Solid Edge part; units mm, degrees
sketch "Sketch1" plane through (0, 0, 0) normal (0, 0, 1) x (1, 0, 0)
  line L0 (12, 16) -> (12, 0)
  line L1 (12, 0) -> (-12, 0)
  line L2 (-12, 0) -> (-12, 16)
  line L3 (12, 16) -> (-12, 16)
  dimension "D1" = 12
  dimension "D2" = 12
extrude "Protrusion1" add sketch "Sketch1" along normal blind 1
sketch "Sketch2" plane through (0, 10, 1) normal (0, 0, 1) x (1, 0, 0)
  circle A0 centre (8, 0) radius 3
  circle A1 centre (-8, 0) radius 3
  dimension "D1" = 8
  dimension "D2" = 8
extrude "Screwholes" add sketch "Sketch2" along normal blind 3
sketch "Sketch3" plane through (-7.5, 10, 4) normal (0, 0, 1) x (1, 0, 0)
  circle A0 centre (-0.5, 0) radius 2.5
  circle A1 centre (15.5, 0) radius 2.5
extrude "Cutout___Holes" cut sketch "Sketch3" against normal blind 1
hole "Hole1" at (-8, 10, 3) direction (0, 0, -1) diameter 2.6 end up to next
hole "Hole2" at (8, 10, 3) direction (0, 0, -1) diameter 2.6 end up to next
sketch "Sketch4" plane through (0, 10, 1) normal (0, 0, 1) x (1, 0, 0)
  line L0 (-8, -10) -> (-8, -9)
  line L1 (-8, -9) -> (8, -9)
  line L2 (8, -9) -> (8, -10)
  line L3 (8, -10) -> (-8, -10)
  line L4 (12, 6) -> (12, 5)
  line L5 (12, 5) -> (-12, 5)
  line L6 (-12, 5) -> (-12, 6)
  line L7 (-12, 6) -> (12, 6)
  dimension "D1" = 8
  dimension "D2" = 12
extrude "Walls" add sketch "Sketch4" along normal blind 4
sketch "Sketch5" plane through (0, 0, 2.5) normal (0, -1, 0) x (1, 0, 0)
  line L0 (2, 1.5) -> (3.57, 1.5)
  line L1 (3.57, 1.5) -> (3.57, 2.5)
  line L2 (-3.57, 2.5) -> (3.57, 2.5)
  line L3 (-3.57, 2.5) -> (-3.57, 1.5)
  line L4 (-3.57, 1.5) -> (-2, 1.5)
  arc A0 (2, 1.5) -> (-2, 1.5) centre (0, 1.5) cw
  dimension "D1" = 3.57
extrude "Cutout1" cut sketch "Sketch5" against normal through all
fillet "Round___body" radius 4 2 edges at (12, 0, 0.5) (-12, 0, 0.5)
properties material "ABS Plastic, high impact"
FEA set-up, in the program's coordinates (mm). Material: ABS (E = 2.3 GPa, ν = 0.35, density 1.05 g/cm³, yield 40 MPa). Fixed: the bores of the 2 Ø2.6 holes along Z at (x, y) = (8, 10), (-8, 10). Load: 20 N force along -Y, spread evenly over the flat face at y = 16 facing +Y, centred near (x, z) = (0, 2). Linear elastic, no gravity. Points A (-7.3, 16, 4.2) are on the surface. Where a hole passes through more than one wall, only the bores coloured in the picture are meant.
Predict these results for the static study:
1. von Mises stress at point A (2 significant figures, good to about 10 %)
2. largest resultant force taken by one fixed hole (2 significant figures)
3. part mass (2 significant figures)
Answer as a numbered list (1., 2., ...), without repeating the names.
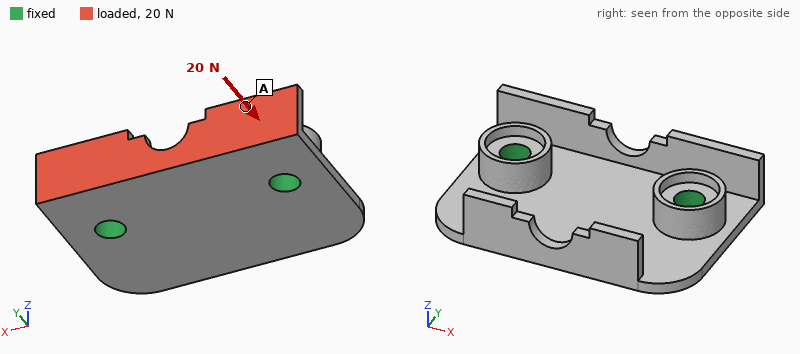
1. 1.0 MPa
2. 10 N
3. 0.64 g
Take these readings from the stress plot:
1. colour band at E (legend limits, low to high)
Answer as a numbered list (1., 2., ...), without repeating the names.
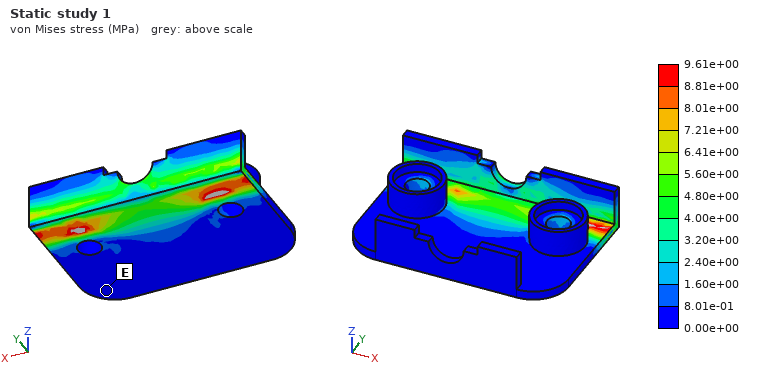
1. 0.00e+00 to 8.01e-01 MPa
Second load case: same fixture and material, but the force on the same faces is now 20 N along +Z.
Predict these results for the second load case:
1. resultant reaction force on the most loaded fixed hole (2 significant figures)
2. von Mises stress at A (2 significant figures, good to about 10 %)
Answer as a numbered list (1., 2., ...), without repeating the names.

1. 10 N
2. 1.4 MPa
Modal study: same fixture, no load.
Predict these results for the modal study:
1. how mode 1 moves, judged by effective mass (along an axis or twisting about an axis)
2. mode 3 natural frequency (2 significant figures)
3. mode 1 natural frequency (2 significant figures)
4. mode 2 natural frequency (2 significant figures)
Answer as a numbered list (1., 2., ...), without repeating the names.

1. along Z
2. 5100 Hz
3. 2400 Hz
4. 4000 Hz
